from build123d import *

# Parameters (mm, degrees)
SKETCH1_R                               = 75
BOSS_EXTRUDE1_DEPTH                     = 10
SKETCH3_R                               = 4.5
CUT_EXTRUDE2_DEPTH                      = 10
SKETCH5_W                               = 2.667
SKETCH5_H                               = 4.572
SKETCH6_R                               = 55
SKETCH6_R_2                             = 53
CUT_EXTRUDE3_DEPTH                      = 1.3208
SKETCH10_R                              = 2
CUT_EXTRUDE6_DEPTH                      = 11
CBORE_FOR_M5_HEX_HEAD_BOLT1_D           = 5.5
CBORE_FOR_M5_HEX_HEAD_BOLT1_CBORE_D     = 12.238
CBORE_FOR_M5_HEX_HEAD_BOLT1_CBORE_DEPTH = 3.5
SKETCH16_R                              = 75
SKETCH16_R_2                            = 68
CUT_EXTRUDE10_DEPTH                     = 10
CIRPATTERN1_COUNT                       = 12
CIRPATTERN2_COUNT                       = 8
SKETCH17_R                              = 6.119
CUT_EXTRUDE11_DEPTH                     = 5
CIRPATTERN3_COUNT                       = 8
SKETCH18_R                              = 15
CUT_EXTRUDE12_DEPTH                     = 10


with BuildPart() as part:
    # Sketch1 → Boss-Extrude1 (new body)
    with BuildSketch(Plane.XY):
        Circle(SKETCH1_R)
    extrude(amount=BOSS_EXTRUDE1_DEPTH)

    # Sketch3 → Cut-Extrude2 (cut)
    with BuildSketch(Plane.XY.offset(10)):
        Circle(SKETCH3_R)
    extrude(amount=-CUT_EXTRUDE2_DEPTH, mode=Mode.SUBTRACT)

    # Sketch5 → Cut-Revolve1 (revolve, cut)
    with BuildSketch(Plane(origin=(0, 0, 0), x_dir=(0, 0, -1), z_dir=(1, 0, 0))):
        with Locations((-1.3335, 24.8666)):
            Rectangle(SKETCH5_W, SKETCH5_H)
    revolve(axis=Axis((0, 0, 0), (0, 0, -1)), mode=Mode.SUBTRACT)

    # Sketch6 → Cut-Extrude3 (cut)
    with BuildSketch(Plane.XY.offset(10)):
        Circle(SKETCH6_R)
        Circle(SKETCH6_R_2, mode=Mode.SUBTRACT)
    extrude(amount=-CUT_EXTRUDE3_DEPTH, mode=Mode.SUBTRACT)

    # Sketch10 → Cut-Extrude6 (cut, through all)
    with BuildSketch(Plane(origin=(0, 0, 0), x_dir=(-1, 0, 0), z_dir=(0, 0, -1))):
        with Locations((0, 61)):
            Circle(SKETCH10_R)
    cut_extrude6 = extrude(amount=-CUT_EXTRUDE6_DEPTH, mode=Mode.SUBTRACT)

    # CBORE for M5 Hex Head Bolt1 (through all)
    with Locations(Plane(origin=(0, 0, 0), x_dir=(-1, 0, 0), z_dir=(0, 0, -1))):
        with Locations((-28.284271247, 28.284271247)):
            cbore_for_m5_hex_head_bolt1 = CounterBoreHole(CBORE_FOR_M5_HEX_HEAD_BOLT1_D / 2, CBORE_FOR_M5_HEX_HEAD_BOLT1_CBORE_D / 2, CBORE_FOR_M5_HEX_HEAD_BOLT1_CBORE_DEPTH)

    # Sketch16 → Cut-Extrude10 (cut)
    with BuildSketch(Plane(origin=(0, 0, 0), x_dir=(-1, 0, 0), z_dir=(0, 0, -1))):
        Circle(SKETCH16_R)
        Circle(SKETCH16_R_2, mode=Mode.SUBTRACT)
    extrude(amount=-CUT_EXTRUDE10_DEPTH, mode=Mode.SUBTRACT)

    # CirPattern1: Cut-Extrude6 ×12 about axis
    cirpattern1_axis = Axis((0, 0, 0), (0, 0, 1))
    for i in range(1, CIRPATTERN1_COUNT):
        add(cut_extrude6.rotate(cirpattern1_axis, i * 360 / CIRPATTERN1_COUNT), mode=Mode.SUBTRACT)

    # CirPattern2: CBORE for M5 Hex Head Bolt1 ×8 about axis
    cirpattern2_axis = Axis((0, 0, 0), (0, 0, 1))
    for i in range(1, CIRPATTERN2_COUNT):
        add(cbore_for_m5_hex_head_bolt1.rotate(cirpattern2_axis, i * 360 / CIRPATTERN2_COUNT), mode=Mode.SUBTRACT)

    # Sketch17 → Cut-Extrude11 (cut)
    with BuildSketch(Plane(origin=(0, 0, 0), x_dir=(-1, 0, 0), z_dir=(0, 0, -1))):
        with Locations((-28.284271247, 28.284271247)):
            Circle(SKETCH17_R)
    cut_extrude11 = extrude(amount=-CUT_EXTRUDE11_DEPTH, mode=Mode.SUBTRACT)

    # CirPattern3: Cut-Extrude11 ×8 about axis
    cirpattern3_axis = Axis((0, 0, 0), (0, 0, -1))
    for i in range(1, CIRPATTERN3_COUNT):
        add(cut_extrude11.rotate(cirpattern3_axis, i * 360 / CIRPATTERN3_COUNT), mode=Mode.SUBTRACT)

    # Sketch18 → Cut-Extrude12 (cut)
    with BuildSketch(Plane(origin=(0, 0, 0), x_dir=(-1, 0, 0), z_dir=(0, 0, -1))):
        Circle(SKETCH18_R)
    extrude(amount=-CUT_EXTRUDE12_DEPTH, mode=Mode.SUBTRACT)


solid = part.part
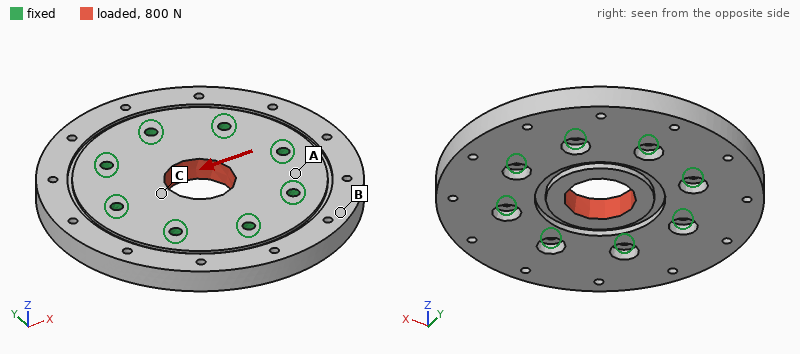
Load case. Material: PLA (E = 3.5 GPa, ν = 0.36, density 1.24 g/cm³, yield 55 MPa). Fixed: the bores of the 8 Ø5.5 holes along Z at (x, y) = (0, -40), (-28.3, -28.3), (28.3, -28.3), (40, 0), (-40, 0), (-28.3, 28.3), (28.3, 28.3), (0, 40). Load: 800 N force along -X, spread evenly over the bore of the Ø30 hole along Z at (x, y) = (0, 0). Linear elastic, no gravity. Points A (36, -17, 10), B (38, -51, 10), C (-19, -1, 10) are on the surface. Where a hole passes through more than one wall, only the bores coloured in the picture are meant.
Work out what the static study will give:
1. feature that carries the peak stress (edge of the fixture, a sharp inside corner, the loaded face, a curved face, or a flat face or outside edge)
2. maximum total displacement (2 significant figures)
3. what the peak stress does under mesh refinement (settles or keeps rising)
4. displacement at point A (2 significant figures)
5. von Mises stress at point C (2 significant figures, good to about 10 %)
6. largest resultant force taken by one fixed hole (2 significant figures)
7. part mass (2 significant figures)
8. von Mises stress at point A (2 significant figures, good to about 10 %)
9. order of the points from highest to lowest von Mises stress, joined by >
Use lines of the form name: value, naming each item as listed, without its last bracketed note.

feature that carries the peak stress: edge of the fixture
maximum total displacement: 11 µm
what the peak stress does under mesh refinement: keeps rising
displacement at point A: 2.6 µm
von Mises stress at point C: 0.75 MPa
largest resultant force taken by one fixed hole: 140 N
part mass: 160 g
von Mises stress at point A: 0.42 MPa
order of the points from highest to lowest von Mises stress, joined by >: C > A > B
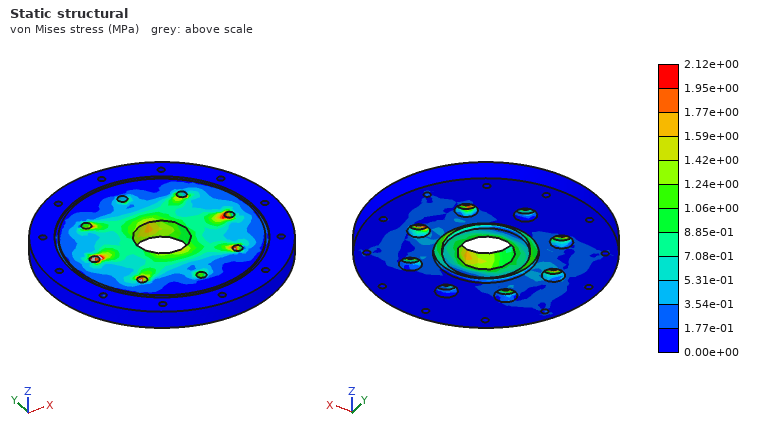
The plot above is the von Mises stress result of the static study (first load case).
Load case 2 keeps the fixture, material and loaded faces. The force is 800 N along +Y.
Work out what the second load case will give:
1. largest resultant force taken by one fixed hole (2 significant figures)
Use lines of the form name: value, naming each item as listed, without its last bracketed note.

largest resultant force taken by one fixed hole: 140 N
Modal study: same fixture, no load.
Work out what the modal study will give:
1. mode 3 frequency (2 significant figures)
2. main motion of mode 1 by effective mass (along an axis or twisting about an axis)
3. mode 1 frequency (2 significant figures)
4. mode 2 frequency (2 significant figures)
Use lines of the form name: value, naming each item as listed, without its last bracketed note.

mode 3 frequency: 2000 Hz
main motion of mode 1 by effective mass: along Z
mode 1 frequency: 1900 Hz
mode 2 frequency: 2000 Hz
